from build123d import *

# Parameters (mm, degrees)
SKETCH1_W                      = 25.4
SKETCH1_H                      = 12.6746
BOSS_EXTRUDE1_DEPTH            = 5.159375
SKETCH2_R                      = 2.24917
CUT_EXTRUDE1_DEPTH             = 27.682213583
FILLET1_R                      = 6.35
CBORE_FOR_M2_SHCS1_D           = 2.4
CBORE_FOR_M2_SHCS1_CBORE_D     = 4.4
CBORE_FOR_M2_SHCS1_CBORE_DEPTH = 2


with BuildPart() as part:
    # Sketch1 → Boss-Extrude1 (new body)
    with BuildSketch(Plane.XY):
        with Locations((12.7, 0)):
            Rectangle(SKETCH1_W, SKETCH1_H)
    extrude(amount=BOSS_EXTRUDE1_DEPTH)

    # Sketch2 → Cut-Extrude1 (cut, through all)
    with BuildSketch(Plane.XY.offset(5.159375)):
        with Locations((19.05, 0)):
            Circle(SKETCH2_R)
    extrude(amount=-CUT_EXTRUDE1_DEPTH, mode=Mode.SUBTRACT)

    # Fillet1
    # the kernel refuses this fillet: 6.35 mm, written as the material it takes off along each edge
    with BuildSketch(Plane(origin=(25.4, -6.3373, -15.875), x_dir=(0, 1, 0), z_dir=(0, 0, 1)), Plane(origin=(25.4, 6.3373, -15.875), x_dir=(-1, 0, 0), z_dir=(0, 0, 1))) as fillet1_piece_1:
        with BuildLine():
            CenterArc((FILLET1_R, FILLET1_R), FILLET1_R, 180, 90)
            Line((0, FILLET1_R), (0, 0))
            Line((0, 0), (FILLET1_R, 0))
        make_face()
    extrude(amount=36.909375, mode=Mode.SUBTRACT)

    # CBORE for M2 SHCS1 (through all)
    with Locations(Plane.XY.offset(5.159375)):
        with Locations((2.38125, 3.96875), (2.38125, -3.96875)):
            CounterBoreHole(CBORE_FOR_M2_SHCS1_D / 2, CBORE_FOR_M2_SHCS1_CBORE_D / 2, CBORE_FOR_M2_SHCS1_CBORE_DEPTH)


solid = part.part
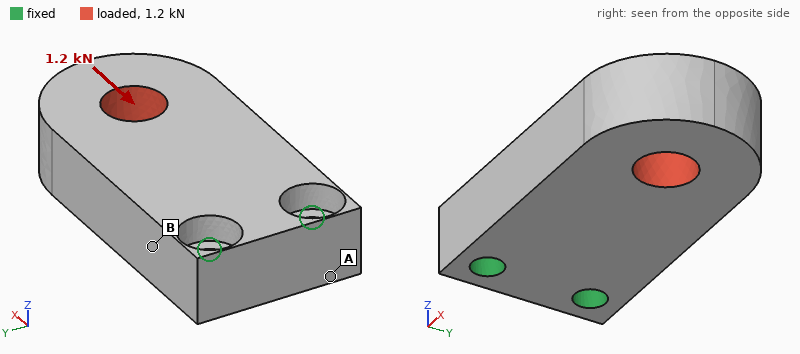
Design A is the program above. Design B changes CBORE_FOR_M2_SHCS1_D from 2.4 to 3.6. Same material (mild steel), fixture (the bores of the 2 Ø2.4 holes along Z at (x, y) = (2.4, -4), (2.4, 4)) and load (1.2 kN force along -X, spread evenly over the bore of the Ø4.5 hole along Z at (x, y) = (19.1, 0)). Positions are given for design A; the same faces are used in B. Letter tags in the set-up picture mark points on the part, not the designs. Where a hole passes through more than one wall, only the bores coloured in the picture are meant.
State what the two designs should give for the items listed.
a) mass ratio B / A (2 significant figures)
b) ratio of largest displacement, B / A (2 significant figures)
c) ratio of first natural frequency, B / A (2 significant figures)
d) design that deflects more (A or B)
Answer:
0.97
0.68
1.2
A
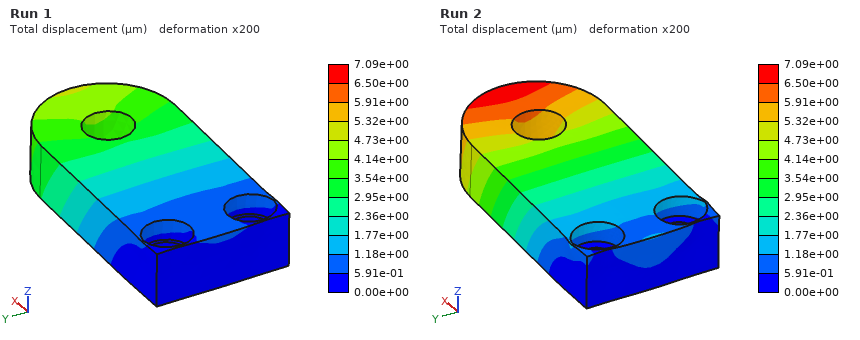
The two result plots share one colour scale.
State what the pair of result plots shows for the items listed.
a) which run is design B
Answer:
Run 1
